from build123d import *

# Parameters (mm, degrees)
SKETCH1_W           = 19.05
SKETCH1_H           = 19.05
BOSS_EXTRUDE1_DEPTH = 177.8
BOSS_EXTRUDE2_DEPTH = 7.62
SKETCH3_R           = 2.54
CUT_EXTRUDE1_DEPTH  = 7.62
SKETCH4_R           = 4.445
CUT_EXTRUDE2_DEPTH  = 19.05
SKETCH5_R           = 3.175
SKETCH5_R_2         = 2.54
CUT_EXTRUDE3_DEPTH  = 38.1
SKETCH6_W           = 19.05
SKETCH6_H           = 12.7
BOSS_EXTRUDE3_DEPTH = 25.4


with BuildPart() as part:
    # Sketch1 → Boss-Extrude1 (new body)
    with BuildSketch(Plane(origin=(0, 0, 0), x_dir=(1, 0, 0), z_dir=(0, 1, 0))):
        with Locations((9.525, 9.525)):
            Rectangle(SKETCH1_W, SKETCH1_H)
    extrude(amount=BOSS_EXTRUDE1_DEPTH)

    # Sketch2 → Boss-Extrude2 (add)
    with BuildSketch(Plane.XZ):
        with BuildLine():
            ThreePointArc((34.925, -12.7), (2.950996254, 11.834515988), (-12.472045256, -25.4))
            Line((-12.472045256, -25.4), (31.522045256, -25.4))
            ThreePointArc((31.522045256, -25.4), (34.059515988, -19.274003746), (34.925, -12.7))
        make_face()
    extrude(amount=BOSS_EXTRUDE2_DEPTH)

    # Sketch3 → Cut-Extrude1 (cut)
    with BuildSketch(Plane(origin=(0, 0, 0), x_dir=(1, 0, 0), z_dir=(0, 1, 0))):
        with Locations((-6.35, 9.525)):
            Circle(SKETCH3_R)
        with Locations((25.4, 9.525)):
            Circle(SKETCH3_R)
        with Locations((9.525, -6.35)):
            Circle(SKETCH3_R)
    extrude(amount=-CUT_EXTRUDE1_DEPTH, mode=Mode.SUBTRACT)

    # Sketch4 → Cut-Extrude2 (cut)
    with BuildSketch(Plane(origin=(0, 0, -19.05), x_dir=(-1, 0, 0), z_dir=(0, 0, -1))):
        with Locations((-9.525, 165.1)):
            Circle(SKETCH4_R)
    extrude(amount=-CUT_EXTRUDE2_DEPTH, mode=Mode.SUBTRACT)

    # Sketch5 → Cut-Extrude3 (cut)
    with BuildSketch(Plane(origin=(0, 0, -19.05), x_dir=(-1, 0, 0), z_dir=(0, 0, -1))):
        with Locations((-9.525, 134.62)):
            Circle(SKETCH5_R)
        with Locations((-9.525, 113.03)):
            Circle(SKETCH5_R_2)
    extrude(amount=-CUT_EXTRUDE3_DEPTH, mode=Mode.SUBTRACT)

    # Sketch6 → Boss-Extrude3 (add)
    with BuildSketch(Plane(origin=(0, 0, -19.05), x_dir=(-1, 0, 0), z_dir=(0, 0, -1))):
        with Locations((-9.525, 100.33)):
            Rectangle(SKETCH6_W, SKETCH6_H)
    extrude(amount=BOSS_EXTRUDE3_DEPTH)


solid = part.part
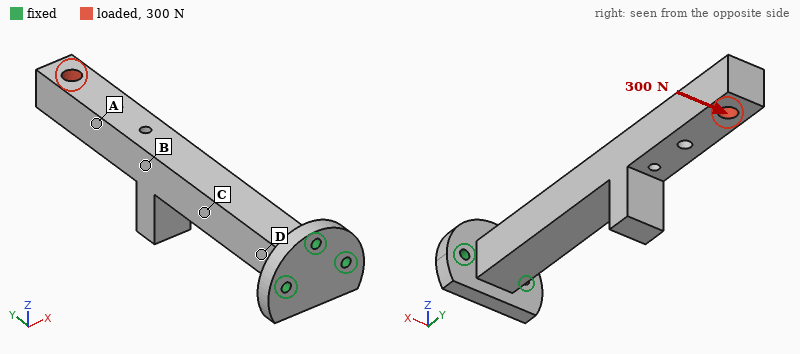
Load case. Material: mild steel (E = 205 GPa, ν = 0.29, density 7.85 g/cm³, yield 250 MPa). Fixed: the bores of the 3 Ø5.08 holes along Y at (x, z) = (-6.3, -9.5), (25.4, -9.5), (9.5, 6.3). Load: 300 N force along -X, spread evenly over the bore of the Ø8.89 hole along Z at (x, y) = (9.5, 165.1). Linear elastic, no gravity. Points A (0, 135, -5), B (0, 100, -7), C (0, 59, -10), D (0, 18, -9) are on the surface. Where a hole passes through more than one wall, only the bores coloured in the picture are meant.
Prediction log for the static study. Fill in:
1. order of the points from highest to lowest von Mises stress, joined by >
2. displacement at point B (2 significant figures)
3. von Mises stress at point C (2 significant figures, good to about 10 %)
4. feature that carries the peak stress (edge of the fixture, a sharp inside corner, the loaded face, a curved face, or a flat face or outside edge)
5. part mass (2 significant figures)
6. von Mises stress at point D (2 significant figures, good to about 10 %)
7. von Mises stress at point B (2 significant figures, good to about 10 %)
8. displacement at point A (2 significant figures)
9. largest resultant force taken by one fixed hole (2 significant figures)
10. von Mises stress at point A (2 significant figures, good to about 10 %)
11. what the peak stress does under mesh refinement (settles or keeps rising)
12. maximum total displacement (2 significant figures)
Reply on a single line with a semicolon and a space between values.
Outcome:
D > C > B > A; 0.11 mm; 28 MPa; edge of the fixture; 630 g; 38 MPa; 17 MPa; 0.17 mm; 1.8 kN; 7.4 MPa; keeps rising; 0.26 mm
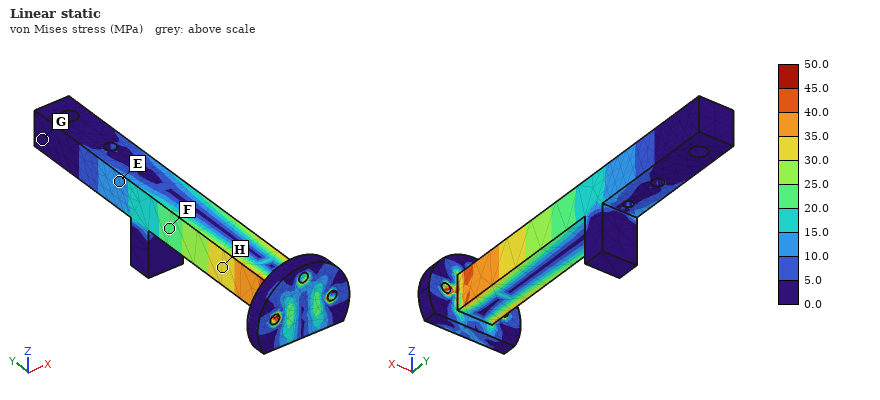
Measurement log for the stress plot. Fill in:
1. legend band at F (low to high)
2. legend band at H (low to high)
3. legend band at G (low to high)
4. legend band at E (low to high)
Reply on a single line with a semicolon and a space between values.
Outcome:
20.0 to 25.0 MPa; 30.0 to 35.0 MPa; 0.0 to 5.0 MPa; 10.0 to 15.0 MPa
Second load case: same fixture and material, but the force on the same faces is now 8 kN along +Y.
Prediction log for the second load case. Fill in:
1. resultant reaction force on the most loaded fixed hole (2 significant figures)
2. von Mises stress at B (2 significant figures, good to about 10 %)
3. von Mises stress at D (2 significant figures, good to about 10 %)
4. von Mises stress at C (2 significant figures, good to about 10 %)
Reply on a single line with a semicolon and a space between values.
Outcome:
3.3 kN; 25 MPa; 22 MPa; 22 MPa
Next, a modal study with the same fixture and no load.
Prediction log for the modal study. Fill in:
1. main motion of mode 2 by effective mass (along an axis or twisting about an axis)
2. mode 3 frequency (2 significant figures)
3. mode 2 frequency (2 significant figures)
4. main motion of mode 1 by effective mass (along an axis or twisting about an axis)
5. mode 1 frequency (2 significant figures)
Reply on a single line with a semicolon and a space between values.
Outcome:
along X; 2400 Hz; 450 Hz; along Z; 420 Hz
